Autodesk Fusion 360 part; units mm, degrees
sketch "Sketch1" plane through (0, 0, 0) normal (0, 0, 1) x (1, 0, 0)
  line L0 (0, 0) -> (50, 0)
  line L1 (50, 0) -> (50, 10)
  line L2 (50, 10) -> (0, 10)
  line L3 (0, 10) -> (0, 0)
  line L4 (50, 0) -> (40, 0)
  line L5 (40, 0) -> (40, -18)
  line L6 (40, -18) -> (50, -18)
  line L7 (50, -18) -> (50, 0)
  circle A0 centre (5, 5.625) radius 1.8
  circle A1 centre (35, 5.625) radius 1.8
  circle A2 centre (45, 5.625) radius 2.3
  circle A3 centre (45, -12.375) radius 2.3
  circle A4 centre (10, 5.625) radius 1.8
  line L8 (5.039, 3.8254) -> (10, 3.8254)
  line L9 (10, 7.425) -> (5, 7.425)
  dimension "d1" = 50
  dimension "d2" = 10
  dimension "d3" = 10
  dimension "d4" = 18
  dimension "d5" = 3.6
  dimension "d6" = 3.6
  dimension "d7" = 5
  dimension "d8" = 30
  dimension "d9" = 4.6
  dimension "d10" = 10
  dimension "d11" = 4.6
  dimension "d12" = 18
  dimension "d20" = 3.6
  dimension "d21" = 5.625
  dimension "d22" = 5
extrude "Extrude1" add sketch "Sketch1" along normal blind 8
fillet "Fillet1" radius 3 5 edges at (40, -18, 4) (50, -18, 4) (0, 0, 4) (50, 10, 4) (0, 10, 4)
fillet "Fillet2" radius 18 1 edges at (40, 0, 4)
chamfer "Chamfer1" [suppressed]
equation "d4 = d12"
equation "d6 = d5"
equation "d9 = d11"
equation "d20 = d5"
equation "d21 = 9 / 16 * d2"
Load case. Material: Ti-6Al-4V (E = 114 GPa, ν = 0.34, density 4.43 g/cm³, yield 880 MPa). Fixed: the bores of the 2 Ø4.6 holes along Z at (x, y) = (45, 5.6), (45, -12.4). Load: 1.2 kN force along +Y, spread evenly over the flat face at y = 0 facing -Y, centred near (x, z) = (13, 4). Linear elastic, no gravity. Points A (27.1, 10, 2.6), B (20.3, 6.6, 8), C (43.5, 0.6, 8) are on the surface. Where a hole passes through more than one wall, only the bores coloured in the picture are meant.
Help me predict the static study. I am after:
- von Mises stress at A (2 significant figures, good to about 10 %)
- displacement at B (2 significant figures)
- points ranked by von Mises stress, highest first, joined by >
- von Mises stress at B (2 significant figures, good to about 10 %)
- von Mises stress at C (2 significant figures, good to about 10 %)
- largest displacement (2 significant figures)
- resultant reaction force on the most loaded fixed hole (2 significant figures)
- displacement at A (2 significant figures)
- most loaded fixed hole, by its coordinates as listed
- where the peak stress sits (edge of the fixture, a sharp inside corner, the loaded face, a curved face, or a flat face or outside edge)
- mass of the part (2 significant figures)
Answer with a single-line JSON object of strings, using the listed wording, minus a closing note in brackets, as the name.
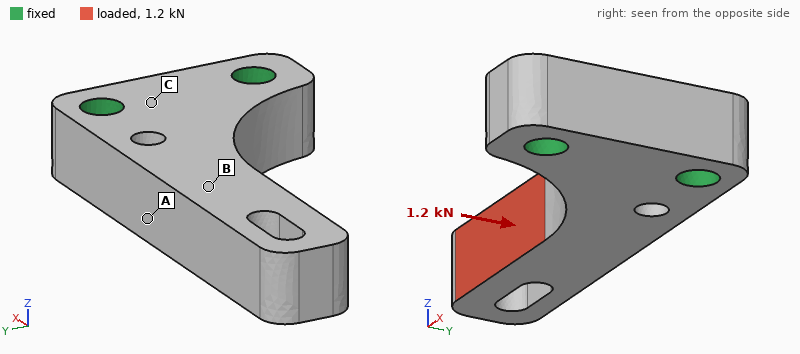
{"von Mises stress at A": "120 MPa", "displacement at B": "0.043 mm", "points ranked by von Mises stress, highest first, joined by >": "A > B > C", "von Mises stress at B": "41 MPa", "von Mises stress at C": "18 MPa", "largest displacement": "0.13 mm", "resultant reaction force on the most loaded fixed hole": "2.3 kN", "displacement at A": "0.026 mm", "most loaded fixed hole, by its coordinates as listed": "(45, -12.4)", "where the peak stress sits": "a curved face", "mass of the part": "24 g"}
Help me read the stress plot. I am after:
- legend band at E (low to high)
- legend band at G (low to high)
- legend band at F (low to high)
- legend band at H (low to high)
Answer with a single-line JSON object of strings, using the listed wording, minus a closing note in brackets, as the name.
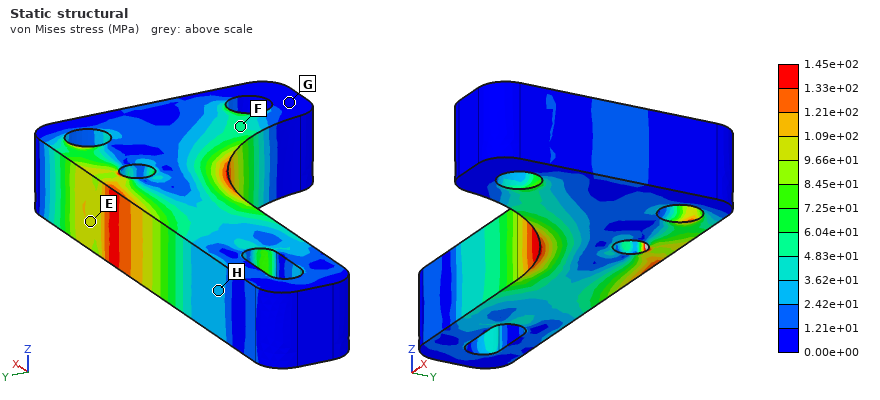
{"legend band at E": "9.66e+01 to 1.09e+02 MPa", "legend band at G": "0.00e+00 to 1.21e+01 MPa", "legend band at F": "4.83e+01 to 6.04e+01 MPa", "legend band at H": "2.42e+01 to 3.62e+01 MPa"}
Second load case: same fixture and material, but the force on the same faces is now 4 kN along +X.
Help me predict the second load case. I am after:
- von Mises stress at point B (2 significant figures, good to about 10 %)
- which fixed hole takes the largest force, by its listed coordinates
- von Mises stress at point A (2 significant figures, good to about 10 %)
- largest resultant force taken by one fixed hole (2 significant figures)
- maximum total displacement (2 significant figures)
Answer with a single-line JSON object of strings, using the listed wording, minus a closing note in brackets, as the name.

{"von Mises stress at point B": "12 MPa", "which fixed hole takes the largest force, by its listed coordinates": "(45, 5.6)", "von Mises stress at point A": "72 MPa", "largest resultant force taken by one fixed hole": "2.8 kN", "maximum total displacement": "0.12 mm"}
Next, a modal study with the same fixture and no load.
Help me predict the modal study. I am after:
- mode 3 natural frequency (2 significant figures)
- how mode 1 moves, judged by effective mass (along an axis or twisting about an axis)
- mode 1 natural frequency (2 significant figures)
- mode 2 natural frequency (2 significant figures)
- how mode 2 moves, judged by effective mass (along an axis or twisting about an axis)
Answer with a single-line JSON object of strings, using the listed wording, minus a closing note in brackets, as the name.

{"mode 3 natural frequency": "18 kHz", "how mode 1 moves, judged by effective mass": "along Z", "mode 1 natural frequency": "4000 Hz", "mode 2 natural frequency": "6700 Hz", "how mode 2 moves, judged by effective mass": "along Y"}
